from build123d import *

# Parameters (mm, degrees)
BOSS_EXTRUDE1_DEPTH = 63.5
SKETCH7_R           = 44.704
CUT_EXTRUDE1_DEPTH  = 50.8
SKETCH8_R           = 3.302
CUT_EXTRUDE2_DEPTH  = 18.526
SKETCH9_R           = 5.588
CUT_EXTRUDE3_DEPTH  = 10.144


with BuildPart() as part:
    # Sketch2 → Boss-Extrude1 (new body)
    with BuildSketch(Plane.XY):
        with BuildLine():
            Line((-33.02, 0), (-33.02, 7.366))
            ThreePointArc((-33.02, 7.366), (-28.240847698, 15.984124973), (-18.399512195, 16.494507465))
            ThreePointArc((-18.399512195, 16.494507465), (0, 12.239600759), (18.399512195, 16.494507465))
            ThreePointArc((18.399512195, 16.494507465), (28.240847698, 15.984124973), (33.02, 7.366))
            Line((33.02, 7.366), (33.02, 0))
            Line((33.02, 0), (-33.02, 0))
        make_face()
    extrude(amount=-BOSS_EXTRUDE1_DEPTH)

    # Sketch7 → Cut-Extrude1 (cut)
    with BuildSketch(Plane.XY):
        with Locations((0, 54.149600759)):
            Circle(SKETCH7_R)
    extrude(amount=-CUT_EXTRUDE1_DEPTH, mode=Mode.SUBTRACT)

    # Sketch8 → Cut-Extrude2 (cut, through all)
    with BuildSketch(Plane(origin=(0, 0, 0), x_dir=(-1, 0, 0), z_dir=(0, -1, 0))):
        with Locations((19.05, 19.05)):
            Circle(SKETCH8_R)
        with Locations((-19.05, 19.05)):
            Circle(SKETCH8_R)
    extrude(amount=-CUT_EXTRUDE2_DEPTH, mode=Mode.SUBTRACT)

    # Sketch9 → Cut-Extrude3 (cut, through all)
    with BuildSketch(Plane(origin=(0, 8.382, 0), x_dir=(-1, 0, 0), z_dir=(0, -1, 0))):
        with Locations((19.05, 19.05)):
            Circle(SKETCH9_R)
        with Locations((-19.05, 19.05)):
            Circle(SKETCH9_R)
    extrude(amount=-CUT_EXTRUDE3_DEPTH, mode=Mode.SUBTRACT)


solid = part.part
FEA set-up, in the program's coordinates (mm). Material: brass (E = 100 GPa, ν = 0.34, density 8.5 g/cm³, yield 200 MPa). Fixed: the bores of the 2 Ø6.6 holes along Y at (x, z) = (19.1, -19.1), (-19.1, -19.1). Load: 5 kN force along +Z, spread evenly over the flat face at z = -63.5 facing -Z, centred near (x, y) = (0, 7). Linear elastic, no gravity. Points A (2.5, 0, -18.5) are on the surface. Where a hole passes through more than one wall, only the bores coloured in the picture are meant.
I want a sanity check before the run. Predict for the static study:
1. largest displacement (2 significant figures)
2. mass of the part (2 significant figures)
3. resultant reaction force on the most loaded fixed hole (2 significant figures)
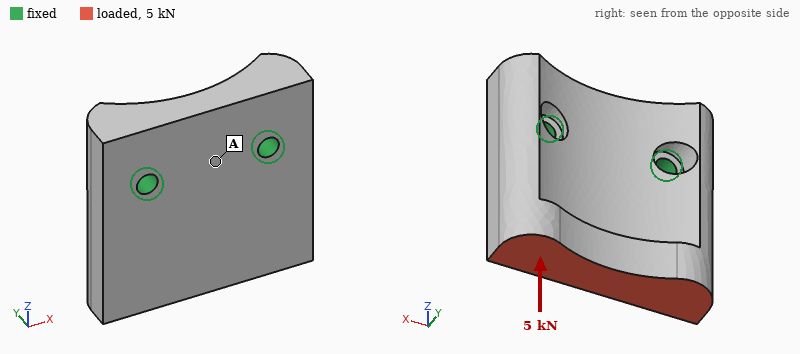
15 µm
450 g
2.5 kN
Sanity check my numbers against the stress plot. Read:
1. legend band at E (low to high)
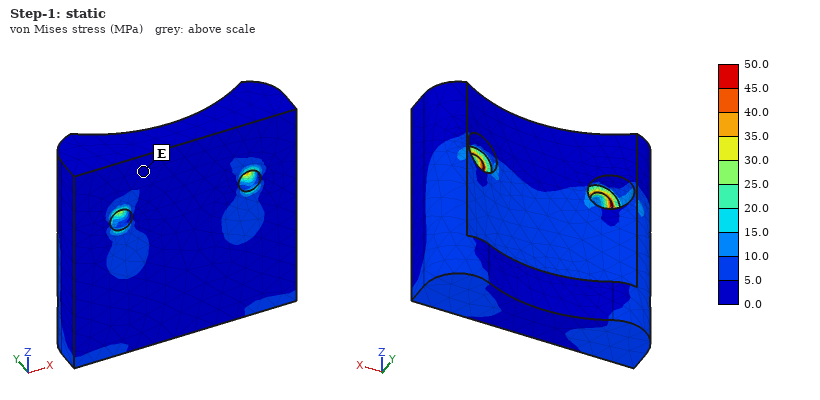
0.0 to 5.0 MPa
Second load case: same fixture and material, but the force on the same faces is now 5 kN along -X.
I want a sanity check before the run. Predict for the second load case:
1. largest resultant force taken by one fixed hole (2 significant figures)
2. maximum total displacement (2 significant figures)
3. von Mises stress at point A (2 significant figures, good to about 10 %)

5.9 kN
24 µm
10 MPa
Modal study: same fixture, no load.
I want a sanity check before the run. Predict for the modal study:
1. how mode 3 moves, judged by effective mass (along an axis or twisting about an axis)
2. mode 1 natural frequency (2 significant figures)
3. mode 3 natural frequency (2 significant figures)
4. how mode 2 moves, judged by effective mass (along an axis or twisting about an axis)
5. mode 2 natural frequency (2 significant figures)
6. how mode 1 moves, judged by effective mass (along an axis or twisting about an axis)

along X
2300 Hz
6800 Hz
twisting about Z
4400 Hz
along Y
